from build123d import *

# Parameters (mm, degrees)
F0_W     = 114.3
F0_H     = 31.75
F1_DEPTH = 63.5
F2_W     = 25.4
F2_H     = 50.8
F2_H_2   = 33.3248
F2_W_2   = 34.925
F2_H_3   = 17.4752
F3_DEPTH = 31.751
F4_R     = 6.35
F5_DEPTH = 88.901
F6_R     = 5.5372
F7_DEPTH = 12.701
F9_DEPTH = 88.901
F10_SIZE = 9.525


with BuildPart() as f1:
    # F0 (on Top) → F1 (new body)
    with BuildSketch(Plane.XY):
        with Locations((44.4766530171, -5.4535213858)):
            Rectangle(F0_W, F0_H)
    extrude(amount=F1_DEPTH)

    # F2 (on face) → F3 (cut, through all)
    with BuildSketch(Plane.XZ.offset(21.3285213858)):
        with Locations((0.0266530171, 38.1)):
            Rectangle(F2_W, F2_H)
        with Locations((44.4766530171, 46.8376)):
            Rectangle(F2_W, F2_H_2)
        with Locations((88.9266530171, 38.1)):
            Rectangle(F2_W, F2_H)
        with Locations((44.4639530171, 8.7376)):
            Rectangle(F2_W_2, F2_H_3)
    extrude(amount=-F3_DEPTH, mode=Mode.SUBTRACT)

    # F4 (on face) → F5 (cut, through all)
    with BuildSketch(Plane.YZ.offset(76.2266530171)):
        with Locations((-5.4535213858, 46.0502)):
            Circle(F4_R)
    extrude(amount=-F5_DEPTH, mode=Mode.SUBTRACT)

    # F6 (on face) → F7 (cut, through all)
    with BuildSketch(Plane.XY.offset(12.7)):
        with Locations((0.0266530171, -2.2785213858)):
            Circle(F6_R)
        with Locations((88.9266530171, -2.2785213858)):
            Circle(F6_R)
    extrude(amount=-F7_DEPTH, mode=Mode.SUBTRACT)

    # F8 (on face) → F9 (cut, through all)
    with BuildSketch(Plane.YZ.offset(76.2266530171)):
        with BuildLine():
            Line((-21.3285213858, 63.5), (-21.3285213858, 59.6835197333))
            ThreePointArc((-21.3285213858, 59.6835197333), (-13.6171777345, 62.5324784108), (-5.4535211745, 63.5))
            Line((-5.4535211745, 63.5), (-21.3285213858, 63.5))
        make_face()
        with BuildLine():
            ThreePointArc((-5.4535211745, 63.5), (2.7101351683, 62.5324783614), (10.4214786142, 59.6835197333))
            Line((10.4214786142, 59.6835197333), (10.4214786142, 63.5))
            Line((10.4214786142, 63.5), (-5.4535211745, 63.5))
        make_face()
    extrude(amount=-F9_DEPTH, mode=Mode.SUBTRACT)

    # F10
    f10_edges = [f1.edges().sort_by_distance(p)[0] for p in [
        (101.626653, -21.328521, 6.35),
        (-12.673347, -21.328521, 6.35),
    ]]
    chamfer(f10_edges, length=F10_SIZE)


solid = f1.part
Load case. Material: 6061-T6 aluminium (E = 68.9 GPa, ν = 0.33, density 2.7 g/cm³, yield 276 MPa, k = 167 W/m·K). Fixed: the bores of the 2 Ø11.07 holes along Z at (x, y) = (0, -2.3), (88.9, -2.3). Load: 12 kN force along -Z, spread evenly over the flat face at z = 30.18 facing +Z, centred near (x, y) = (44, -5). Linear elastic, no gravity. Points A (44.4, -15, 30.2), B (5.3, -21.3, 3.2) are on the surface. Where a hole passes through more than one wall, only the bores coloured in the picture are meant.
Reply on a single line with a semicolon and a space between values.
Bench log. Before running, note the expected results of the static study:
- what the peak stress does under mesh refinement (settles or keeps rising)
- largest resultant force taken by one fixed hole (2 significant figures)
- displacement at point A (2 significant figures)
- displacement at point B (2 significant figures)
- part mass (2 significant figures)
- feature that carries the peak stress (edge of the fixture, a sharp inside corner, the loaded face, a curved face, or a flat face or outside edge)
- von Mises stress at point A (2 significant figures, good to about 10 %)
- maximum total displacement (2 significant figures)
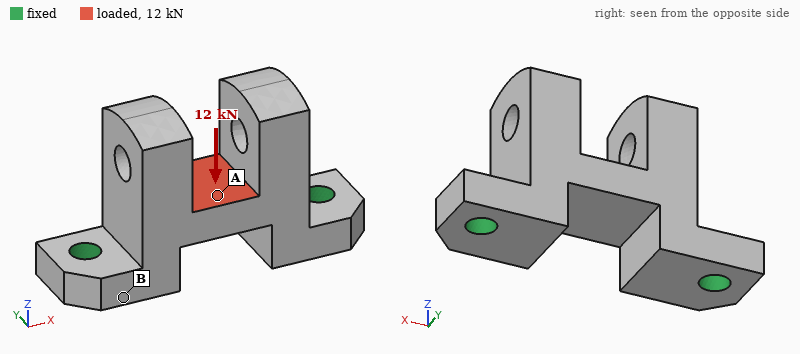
keeps rising; 9.0 kN; 54 µm; 14 µm; 250 g; edge of the fixture; 61 MPa; 64 µm
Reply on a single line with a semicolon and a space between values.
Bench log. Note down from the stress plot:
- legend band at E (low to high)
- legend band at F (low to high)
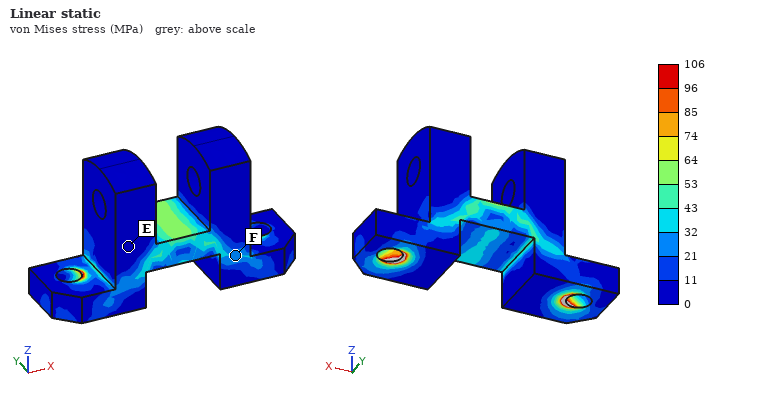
0 to 11 MPa; 21 to 32 MPa
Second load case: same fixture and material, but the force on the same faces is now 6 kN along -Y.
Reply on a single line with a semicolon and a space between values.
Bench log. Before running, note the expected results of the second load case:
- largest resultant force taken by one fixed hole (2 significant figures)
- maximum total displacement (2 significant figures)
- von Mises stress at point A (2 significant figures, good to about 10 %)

3.0 kN; 0.14 mm; 15 MPa
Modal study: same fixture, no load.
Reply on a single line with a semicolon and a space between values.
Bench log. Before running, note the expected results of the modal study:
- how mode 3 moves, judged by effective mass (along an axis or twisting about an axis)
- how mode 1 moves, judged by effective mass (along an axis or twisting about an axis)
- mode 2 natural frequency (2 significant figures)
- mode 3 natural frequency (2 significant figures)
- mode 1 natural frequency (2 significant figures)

along X; along Y; 4500 Hz; 5700 Hz; 2700 Hz
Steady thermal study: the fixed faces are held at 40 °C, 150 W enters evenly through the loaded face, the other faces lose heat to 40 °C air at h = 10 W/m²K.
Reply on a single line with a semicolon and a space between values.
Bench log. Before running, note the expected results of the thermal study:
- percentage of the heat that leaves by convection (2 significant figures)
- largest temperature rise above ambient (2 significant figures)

3.1 %; 48 K
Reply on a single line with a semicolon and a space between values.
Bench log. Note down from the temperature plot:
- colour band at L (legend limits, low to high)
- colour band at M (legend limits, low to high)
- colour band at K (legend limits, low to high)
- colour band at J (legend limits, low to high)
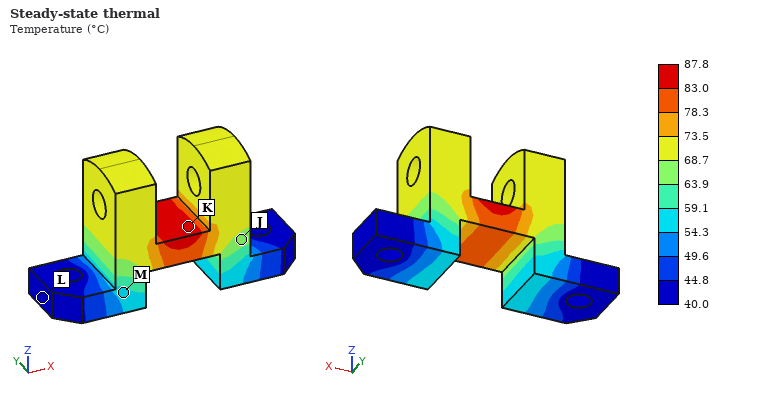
40.0 to 44.8 °C; 54.3 to 59.1 °C; 83.0 to 87.8 °C; 63.9 to 68.7 °C
